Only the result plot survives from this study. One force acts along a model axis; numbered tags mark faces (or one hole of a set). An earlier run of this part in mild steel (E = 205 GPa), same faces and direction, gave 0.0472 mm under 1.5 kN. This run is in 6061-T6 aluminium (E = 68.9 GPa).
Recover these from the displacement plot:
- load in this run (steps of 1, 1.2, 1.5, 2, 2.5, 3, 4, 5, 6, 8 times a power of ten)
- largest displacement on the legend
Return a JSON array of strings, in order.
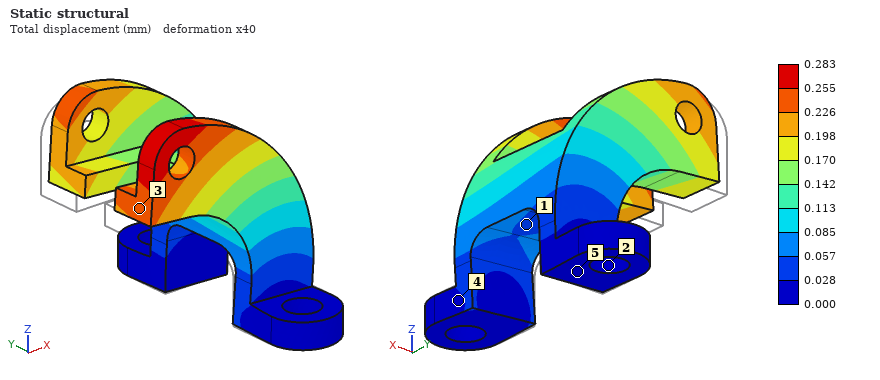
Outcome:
["3 kN", "0.283 mm"]
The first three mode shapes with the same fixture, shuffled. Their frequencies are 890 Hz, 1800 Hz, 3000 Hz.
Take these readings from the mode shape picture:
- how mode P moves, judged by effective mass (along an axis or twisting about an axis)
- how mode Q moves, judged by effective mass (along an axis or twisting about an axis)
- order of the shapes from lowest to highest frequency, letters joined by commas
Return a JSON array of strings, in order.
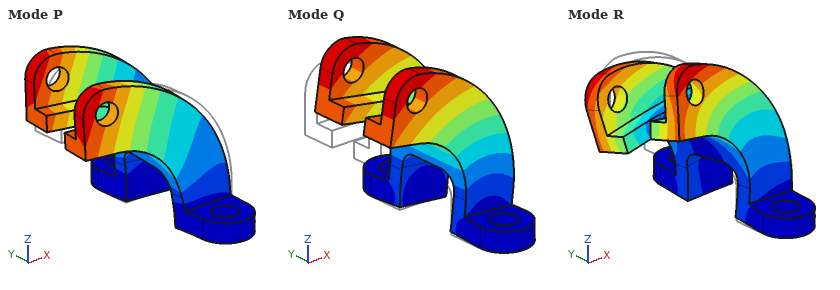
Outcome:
["along Y", "along X", "Q, P, R"]
